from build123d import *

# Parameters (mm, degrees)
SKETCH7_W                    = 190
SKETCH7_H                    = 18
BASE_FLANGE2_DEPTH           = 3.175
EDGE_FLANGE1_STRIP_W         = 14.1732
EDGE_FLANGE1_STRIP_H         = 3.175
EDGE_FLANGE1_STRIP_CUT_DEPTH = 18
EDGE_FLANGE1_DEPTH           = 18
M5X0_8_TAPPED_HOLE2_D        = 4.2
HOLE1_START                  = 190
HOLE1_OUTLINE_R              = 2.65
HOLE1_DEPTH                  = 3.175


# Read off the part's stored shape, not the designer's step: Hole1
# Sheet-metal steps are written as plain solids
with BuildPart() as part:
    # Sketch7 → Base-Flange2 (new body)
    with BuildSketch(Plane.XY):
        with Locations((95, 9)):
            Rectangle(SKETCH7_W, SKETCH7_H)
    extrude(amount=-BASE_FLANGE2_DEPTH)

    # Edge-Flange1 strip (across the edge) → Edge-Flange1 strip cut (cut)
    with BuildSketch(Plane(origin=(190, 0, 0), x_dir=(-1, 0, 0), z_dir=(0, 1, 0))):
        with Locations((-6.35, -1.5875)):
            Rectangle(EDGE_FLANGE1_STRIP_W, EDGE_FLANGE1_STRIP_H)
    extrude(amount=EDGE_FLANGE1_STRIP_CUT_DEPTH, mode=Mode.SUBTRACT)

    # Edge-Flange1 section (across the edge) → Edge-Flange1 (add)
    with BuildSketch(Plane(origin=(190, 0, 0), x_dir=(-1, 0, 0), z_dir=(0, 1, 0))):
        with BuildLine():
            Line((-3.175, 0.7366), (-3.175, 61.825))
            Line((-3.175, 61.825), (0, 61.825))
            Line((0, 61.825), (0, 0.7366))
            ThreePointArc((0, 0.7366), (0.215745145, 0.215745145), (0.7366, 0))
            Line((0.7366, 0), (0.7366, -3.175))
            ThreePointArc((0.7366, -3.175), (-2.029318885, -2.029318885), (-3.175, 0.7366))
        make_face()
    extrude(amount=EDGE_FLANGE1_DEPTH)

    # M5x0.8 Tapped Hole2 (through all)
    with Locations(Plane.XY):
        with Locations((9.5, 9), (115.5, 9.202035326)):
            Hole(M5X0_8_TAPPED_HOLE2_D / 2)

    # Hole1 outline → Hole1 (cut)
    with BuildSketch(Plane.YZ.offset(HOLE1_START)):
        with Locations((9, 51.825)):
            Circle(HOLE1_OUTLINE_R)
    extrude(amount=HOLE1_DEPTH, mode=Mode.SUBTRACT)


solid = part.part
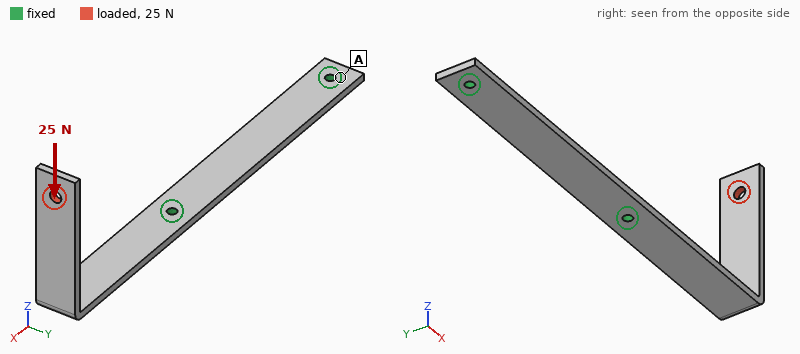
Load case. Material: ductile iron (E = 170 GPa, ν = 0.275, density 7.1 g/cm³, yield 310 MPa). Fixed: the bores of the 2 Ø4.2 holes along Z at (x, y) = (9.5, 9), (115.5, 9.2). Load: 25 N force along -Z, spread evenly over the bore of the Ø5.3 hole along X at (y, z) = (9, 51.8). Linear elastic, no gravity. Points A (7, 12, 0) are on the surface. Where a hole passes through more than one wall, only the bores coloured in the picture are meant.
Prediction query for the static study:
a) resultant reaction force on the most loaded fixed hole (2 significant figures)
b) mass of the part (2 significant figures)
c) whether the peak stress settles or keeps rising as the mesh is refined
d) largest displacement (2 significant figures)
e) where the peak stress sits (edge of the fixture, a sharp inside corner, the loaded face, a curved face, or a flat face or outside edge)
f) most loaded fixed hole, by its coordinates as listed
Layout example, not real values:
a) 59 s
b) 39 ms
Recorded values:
a) 25 N
b) 100 g
c) keeps rising
d) 0.71 mm
e) edge of the fixture
f) (115.5, 9.2)
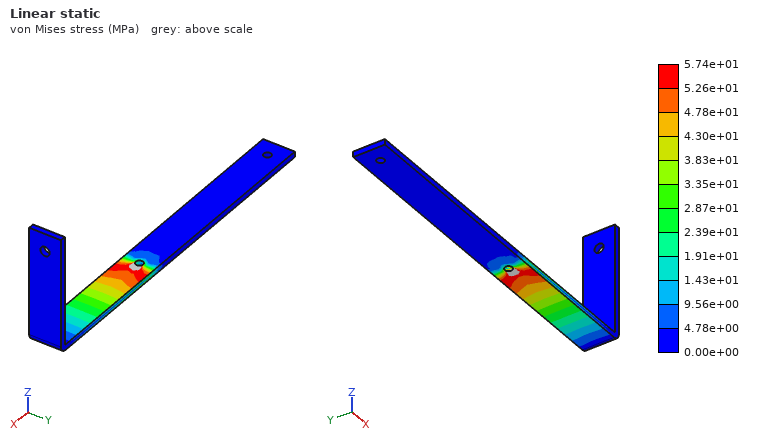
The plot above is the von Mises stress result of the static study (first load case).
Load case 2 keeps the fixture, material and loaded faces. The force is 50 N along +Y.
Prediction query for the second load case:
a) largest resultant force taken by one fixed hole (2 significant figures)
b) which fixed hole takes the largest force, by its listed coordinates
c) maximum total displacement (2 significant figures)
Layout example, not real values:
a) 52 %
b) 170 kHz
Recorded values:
a) 68 N
b) (115.5, 9.2)
c) 1.1 mm
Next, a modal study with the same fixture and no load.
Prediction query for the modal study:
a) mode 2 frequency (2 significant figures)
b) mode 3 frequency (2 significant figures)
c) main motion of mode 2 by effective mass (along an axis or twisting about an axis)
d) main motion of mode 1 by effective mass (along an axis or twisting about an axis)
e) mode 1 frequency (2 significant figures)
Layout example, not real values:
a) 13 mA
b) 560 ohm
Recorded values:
a) 330 Hz
b) 510 Hz
c) along Y
d) along Z
e) 180 Hz
